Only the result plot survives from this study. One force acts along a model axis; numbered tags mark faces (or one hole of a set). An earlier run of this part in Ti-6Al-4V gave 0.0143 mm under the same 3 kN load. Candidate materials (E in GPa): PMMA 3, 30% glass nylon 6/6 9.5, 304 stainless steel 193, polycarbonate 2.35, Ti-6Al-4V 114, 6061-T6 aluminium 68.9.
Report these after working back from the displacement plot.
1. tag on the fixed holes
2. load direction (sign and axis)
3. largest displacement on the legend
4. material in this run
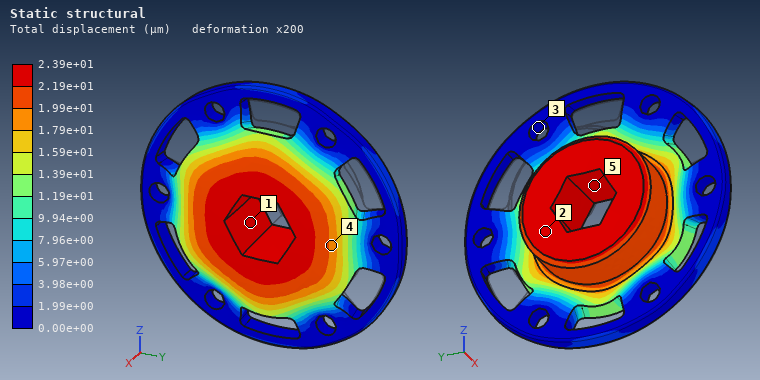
3
+X
2.39e+01 µm
6061-T6 aluminium
